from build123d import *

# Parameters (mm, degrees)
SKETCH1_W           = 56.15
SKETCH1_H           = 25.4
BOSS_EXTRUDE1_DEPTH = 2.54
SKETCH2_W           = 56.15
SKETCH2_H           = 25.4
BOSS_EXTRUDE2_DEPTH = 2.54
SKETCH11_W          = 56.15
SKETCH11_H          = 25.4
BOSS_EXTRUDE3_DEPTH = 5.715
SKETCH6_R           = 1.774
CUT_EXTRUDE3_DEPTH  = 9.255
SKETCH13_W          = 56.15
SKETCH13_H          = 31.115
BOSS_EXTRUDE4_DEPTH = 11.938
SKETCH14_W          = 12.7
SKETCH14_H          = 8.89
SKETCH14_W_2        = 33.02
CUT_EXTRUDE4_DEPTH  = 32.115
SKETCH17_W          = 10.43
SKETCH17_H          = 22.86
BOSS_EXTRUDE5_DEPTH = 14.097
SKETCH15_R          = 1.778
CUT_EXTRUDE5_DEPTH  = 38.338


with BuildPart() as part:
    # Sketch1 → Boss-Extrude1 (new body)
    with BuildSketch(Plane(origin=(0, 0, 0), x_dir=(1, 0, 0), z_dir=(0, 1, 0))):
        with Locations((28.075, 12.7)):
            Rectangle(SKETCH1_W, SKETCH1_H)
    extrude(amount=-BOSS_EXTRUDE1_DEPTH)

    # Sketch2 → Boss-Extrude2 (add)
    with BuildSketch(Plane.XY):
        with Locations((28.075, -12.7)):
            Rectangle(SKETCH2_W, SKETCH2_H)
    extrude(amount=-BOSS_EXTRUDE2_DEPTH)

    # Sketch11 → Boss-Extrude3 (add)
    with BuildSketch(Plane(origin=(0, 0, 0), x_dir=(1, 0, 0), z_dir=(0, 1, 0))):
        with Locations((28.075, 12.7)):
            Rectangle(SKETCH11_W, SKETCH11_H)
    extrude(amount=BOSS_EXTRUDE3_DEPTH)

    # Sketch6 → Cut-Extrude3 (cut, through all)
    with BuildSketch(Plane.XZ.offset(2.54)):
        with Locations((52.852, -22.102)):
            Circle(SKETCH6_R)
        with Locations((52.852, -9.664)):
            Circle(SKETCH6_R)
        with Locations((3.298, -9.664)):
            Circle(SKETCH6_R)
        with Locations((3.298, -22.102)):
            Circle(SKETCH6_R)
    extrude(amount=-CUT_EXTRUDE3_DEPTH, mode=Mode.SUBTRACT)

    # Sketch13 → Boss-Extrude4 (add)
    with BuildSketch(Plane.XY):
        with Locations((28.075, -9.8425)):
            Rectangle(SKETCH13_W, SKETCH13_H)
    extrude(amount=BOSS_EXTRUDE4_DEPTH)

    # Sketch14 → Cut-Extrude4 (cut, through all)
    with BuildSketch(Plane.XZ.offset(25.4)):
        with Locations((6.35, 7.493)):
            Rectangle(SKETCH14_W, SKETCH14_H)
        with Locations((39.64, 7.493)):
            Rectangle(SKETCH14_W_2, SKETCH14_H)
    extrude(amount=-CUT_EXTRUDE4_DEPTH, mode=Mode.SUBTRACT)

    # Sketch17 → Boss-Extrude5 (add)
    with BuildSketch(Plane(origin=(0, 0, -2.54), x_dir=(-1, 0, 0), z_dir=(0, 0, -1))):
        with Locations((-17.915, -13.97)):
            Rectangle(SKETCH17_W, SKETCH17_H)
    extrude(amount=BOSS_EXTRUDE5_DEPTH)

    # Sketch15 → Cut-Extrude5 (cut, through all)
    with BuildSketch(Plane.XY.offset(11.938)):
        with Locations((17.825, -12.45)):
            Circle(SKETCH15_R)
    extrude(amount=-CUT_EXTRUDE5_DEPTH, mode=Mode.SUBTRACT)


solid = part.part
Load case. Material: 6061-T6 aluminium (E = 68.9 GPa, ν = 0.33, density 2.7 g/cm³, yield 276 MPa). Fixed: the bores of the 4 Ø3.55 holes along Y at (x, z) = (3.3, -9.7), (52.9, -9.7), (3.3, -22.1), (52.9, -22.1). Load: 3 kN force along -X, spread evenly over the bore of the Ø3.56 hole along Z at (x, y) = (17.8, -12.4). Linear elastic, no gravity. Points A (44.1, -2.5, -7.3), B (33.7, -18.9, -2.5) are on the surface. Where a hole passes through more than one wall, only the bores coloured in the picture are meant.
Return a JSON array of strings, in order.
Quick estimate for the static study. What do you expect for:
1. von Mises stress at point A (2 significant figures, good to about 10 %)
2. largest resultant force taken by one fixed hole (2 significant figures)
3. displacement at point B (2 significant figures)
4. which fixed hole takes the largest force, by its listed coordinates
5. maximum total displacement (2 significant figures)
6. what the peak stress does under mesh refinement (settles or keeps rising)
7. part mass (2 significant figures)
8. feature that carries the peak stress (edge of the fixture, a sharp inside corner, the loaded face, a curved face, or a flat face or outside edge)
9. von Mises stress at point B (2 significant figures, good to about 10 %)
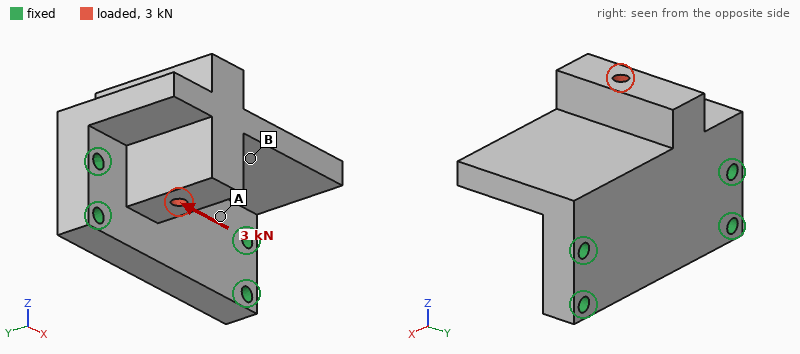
["19 MPa", "1.6 kN", "12 µm", "(3.3, -9.7)", "20 µm", "keeps rising", "70 g", "edge of the fixture", "8.7 MPa"]
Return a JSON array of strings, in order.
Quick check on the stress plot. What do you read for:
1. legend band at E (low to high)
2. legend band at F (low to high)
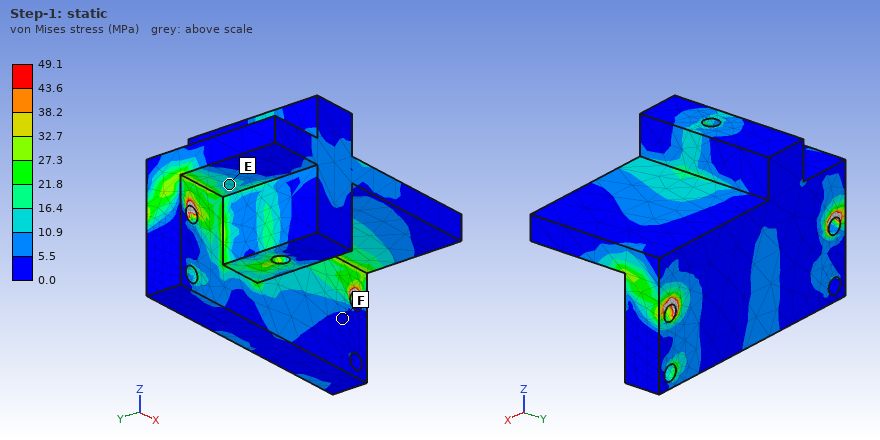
["10.9 to 16.4 MPa", "0.0 to 5.5 MPa"]
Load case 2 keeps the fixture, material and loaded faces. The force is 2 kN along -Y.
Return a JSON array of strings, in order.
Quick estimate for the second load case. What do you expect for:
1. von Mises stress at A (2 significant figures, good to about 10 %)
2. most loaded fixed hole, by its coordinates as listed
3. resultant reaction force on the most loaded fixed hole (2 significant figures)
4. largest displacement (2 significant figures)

["9.2 MPa", "(3.3, -9.7)", "1.6 kN", "31 µm"]
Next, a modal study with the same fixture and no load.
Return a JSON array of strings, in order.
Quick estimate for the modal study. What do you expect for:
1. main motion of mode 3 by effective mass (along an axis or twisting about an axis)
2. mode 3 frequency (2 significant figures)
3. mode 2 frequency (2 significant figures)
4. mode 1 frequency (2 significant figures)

["along Y", "12 kHz", "9300 Hz", "5500 Hz"]
